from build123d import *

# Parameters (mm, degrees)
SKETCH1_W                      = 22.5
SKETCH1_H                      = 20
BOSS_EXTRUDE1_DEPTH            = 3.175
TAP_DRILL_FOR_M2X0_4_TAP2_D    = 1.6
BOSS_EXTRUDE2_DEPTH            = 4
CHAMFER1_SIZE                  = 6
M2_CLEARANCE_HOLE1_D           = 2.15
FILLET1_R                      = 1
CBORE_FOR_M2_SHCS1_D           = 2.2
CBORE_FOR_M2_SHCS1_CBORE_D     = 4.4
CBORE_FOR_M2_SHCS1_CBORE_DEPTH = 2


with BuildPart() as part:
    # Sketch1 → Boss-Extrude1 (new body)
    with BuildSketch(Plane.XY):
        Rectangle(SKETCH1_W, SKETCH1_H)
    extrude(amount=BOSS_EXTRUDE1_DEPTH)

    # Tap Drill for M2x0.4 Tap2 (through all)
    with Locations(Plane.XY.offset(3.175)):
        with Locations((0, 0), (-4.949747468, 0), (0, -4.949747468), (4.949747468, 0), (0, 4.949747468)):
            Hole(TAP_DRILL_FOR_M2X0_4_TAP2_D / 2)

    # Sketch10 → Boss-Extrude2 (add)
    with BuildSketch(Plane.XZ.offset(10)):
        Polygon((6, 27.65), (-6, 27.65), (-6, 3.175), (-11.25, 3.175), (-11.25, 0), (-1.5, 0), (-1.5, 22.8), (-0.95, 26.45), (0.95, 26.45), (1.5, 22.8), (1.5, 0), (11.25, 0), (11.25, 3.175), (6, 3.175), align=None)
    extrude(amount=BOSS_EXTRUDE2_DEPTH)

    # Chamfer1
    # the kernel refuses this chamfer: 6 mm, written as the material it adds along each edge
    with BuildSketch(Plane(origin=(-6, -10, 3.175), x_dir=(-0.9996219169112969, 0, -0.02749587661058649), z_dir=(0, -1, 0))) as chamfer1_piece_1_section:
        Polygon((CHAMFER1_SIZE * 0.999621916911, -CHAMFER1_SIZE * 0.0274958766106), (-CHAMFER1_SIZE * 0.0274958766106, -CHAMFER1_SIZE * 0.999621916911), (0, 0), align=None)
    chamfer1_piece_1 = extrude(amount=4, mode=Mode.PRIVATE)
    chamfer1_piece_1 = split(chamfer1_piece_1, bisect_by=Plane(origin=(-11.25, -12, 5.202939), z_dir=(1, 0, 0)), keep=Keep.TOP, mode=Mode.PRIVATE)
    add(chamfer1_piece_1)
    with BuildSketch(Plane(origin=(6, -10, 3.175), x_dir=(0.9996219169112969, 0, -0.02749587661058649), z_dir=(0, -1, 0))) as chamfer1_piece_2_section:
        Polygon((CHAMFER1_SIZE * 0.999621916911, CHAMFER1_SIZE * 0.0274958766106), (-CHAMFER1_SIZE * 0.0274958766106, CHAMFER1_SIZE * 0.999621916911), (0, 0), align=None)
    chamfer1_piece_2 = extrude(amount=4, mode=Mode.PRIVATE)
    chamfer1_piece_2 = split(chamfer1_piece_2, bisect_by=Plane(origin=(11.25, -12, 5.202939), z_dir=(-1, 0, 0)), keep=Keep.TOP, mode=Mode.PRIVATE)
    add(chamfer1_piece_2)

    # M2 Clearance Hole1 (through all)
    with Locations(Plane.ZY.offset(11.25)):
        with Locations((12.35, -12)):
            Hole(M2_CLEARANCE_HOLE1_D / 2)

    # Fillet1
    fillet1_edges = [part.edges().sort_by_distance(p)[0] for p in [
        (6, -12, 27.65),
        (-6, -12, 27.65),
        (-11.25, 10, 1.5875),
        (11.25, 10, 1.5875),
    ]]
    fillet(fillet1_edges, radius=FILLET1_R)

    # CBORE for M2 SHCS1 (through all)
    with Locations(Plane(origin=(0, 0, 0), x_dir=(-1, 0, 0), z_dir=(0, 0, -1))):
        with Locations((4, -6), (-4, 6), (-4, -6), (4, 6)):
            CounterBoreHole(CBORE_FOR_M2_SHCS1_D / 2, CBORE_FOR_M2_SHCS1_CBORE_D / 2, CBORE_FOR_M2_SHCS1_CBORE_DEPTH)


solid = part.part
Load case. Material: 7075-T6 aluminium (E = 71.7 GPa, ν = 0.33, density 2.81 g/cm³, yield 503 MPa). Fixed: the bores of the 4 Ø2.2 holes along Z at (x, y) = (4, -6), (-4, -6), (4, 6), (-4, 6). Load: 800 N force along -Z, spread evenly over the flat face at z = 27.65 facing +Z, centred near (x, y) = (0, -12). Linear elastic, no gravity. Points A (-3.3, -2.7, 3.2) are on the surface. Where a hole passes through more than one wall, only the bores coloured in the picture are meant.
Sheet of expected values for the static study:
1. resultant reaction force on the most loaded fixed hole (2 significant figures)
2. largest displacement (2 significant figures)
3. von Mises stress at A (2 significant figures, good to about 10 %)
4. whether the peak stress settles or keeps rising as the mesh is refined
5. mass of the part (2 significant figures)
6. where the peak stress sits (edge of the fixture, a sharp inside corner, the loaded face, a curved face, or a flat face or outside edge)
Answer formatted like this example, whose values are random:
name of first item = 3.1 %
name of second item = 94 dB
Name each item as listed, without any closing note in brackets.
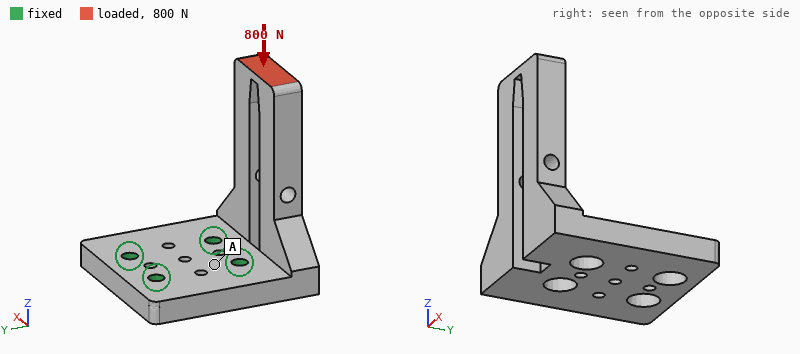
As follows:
resultant reaction force on the most loaded fixed hole = 610 N
largest displacement = 0.20 mm
von Mises stress at A = 26 MPa
whether the peak stress settles or keeps rising as the mesh is refined = keeps rising
mass of the part = 7.1 g
where the peak stress sits = edge of the fixture
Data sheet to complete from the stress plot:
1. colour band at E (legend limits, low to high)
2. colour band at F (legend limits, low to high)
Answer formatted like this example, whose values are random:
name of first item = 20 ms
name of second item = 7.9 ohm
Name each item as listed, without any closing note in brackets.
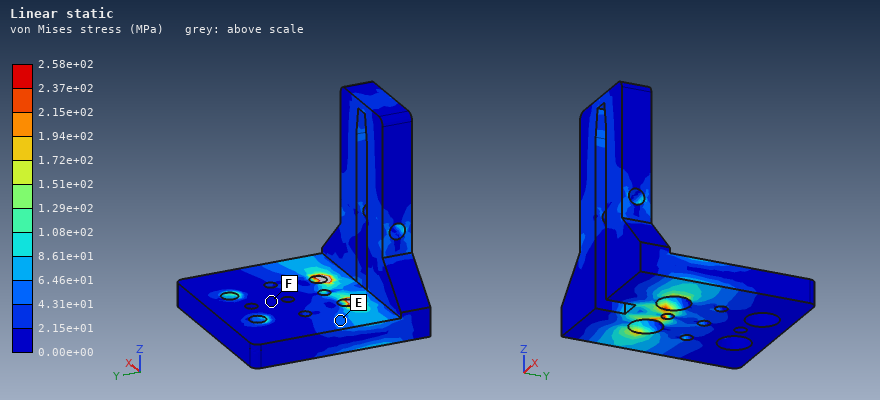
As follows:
colour band at E = 4.31e+01 to 6.46e+01 MPa
colour band at F = 0.00e+00 to 2.15e+01 MPa
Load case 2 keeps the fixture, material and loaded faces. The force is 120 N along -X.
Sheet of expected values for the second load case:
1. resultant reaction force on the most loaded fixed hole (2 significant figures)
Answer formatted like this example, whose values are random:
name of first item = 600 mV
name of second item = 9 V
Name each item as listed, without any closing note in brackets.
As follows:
resultant reaction force on the most loaded fixed hole = 330 N
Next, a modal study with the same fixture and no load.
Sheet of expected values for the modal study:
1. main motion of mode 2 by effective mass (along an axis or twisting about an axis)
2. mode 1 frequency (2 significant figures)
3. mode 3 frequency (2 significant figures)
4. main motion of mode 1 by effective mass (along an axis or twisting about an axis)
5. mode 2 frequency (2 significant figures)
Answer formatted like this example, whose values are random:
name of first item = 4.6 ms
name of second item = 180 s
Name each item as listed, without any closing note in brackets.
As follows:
main motion of mode 2 by effective mass = along X
mode 1 frequency = 3400 Hz
mode 3 frequency = 12 kHz
main motion of mode 1 by effective mass = along Y
mode 2 frequency = 5600 Hz
